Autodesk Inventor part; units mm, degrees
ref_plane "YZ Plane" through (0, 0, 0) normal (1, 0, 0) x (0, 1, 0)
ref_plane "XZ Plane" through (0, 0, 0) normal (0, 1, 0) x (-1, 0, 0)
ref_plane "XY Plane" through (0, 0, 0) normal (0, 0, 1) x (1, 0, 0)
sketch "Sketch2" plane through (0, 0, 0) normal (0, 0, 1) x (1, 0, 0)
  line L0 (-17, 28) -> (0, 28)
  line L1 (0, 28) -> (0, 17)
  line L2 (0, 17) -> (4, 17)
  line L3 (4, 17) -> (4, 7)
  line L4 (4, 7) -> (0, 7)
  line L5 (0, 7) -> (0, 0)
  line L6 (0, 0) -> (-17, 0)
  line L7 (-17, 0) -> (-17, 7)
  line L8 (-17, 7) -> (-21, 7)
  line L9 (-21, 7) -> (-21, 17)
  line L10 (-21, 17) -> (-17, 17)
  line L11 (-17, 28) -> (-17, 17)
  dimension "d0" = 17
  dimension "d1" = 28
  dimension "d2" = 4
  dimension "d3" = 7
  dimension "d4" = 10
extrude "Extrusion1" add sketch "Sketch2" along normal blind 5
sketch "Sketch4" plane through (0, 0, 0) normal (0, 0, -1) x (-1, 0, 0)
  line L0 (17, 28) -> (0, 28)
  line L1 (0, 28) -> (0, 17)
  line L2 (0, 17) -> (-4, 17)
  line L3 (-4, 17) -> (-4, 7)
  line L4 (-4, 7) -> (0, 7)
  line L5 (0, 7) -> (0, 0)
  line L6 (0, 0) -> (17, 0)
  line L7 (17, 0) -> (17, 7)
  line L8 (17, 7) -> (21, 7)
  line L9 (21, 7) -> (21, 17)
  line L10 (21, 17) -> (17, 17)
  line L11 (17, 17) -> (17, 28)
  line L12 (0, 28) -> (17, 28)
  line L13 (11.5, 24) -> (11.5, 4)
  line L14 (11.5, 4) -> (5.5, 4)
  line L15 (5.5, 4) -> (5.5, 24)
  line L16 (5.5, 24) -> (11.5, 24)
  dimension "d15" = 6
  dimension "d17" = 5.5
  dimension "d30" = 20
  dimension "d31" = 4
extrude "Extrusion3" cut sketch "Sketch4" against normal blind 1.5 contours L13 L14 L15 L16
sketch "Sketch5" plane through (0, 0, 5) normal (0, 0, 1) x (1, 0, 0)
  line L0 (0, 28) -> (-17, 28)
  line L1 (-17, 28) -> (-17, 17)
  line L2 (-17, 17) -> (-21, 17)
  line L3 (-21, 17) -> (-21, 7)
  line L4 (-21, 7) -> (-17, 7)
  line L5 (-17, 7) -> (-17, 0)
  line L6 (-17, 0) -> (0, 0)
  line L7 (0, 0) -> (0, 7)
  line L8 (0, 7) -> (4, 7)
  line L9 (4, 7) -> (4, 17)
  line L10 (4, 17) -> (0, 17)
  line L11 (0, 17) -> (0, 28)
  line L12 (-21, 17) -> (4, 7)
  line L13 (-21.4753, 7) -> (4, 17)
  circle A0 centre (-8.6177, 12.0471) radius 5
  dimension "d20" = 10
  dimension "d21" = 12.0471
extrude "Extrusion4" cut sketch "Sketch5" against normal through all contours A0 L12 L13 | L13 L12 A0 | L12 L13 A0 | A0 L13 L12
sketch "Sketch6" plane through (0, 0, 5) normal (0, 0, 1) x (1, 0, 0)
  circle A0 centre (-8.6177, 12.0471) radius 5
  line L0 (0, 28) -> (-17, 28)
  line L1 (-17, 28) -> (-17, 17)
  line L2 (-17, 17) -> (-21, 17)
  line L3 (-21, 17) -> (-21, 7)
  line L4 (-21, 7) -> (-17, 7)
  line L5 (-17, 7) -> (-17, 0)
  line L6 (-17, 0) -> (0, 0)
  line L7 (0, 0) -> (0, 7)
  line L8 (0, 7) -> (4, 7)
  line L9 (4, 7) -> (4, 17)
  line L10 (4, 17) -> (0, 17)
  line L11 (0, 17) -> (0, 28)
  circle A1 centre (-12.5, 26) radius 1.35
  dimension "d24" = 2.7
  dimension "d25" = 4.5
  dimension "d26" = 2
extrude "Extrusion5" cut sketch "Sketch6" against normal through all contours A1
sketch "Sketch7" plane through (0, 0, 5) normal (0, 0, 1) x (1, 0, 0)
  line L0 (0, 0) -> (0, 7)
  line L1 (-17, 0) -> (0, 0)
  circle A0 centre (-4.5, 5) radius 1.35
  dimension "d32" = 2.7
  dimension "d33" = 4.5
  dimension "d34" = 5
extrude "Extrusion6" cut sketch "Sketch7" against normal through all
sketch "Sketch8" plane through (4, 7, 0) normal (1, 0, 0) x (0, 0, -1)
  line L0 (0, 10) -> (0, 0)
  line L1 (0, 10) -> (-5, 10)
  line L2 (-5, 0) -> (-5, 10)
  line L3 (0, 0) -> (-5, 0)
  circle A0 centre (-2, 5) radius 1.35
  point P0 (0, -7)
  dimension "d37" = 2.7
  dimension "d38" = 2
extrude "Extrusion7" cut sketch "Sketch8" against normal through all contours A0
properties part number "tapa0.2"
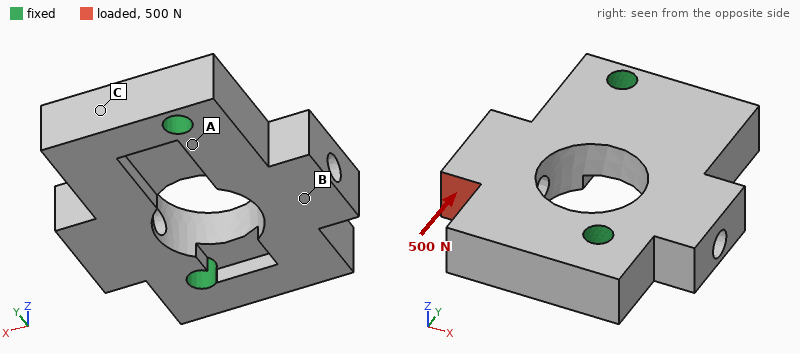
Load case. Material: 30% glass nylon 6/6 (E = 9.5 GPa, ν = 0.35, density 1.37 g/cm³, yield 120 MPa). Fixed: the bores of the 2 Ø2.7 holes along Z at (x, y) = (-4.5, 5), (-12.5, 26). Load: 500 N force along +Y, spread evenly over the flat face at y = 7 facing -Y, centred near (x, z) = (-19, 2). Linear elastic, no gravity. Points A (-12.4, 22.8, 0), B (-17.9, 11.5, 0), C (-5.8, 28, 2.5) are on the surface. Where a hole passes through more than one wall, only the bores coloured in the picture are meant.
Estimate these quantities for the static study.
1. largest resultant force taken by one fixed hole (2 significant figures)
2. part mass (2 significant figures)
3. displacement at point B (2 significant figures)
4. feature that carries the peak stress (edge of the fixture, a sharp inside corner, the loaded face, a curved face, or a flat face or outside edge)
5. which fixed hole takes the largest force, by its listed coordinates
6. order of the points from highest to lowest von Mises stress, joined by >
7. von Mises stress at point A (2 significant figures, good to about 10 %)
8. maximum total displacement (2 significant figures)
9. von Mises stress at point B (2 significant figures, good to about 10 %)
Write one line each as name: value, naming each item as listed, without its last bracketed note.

largest resultant force taken by one fixed hole: 410 N
part mass: 2.9 g
displacement at point B: 32 µm
feature that carries the peak stress: a curved face
which fixed hole takes the largest force, by its listed coordinates: (-12.5, 26)
order of the points from highest to lowest von Mises stress, joined by >: B > A > C
von Mises stress at point A: 14 MPa
maximum total displacement: 60 µm
von Mises stress at point B: 35 MPa
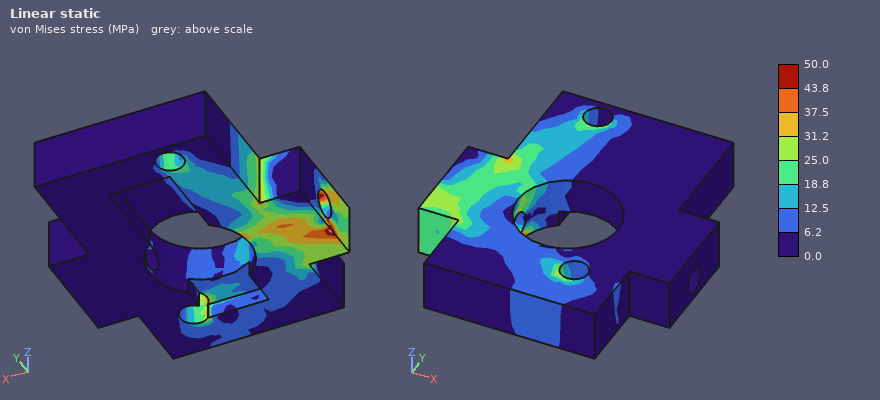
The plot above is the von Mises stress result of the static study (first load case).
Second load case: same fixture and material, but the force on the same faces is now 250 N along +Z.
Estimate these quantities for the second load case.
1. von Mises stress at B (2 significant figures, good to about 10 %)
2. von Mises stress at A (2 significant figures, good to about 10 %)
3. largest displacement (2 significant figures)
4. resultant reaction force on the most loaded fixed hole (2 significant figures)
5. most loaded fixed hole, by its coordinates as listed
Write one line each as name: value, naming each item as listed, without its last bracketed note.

von Mises stress at B: 51 MPa
von Mises stress at A: 47 MPa
largest displacement: 0.35 mm
resultant reaction force on the most loaded fixed hole: 160 N
most loaded fixed hole, by its coordinates as listed: (-4.5, 5)
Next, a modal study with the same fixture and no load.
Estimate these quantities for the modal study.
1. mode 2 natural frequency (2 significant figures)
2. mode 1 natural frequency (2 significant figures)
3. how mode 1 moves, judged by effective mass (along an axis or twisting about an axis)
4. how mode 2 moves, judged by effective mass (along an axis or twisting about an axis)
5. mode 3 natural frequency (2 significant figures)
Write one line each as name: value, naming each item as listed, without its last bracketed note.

mode 2 natural frequency: 11 kHz
mode 1 natural frequency: 8200 Hz
how mode 1 moves, judged by effective mass: along Z
how mode 2 moves, judged by effective mass: along Z
mode 3 natural frequency: 18 kHz
